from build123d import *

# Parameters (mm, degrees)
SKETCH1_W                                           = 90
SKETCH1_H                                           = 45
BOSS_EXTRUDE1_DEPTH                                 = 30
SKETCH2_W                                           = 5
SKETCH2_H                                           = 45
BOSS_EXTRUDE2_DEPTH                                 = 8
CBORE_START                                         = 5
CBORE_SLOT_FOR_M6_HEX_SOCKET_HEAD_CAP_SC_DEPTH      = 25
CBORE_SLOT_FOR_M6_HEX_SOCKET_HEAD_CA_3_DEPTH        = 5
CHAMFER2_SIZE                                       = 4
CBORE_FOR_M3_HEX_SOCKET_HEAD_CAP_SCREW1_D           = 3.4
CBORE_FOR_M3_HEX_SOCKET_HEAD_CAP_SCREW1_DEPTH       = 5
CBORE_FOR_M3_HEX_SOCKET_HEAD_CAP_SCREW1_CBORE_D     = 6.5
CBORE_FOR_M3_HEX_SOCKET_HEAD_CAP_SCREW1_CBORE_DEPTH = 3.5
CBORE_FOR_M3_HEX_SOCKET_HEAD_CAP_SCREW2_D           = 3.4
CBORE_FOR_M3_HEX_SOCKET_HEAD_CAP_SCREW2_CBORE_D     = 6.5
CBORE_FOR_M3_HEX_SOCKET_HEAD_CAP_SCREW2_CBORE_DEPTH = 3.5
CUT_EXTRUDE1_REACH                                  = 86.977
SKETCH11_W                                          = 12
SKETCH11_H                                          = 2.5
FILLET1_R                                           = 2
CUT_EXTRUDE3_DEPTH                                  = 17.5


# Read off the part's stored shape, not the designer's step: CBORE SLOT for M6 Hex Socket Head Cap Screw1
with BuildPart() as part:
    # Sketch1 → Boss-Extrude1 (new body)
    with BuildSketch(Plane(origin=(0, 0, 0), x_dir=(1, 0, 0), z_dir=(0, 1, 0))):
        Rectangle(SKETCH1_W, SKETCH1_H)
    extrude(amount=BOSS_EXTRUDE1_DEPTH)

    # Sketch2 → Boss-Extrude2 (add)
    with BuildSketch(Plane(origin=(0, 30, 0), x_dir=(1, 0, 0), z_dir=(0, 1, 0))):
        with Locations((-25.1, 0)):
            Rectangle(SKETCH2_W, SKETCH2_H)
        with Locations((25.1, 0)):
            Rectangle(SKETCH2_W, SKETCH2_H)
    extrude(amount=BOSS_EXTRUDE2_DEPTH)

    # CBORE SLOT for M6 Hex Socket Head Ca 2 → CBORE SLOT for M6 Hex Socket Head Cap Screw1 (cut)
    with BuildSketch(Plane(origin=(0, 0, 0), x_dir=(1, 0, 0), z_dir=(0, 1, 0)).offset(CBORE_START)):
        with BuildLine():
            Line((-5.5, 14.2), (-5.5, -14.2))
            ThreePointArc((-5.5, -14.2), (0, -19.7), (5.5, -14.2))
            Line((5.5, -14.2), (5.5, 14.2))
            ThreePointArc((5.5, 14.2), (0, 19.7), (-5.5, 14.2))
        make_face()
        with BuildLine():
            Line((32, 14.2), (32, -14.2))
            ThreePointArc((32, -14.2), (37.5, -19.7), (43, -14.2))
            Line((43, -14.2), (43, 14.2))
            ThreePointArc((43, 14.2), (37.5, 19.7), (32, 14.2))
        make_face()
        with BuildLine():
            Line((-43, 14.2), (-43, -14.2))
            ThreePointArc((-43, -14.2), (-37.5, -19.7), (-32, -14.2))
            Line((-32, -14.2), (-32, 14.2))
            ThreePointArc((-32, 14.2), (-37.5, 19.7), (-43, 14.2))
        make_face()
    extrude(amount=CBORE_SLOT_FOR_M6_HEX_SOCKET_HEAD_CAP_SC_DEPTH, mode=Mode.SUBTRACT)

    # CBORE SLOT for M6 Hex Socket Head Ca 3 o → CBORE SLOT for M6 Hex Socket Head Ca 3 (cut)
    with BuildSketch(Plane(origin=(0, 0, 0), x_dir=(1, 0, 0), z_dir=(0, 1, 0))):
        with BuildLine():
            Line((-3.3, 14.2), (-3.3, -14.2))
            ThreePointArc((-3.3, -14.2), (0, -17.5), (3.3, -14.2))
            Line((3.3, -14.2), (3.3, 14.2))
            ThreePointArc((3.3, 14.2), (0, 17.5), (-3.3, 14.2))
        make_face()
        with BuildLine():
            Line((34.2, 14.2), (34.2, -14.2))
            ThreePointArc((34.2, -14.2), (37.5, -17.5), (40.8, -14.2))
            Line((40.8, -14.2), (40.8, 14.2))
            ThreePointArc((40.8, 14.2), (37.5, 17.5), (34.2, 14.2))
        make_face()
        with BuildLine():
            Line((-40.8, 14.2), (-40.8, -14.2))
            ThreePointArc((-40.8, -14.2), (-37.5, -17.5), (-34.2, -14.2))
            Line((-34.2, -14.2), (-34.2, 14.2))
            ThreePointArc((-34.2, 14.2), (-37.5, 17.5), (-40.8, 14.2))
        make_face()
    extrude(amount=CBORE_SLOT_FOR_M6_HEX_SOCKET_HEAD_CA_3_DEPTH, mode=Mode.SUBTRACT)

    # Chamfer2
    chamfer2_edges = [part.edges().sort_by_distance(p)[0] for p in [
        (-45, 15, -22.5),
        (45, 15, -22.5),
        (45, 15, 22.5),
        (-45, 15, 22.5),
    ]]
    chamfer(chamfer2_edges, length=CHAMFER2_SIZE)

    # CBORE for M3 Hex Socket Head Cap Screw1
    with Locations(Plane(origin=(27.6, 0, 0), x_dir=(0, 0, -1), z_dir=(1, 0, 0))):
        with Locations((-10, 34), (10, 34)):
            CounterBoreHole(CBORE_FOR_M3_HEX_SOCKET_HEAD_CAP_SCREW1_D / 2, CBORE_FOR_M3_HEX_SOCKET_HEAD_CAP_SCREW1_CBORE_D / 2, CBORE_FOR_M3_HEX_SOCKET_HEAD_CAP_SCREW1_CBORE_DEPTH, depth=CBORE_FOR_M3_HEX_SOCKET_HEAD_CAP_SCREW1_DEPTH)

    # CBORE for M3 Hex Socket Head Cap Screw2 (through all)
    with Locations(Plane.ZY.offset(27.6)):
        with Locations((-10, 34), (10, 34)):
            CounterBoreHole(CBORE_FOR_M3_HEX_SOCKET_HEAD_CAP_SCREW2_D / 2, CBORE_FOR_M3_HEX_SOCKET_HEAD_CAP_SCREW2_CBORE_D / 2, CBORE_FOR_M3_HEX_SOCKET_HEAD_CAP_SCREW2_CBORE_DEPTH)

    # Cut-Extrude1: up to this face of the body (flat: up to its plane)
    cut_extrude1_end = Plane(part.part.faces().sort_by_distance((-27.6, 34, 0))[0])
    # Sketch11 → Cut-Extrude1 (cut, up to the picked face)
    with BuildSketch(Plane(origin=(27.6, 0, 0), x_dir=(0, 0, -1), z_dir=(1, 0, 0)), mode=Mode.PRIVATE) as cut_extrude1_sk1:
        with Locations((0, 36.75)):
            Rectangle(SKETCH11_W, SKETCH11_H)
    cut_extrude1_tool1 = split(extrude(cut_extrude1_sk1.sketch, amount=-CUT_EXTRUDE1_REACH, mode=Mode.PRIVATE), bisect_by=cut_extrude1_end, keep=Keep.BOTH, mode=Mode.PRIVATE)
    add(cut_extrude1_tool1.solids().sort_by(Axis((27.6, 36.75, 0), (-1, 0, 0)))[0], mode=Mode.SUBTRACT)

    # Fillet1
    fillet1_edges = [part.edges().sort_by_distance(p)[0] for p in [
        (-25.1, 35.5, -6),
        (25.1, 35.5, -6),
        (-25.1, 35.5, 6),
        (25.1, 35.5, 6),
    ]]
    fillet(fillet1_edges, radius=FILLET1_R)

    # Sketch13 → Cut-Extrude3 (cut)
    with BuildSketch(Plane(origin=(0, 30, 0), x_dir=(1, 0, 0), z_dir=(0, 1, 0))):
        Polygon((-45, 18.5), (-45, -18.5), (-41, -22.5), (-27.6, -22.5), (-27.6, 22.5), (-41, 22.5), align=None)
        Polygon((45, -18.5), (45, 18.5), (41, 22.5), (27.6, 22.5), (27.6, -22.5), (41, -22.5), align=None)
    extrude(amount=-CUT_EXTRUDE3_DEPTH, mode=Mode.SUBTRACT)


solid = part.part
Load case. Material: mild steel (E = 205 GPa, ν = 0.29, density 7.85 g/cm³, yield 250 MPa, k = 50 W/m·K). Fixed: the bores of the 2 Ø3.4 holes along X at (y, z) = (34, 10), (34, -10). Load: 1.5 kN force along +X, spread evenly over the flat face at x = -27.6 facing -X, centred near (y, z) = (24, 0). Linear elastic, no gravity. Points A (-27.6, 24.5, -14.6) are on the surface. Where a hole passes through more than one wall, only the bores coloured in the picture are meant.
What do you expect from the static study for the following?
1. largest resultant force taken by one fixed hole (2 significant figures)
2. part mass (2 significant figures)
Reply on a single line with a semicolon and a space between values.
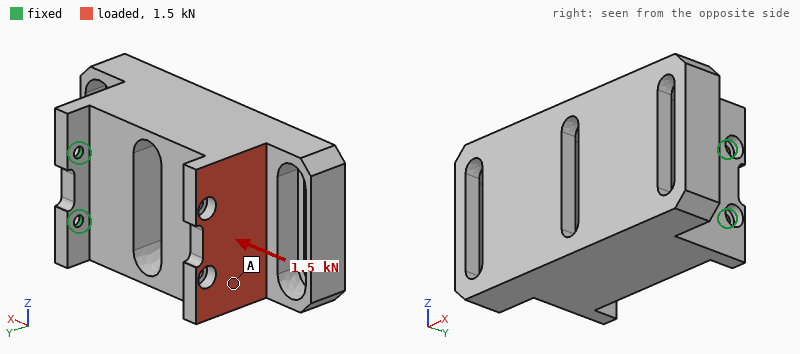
750 N; 600 g
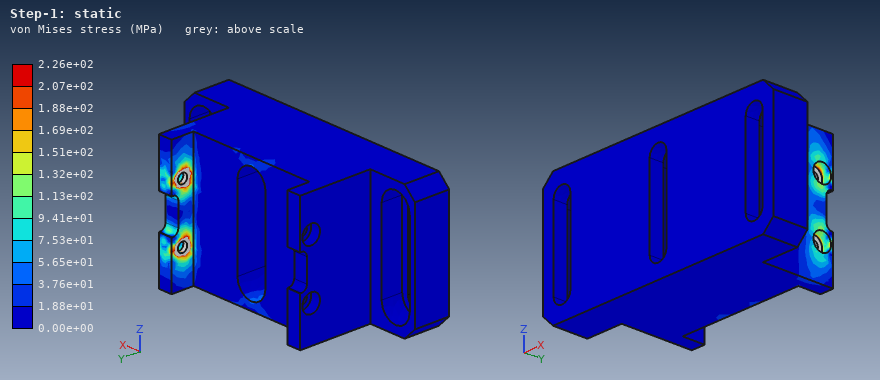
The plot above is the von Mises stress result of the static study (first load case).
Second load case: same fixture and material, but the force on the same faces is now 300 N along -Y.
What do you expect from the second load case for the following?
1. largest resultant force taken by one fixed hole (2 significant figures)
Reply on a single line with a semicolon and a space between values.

150 N
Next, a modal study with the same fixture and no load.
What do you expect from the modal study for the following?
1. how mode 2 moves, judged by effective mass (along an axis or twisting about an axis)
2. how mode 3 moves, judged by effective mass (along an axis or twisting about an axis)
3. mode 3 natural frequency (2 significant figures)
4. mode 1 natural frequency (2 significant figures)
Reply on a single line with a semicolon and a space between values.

along Z; along Z; 3200 Hz; 270 Hz
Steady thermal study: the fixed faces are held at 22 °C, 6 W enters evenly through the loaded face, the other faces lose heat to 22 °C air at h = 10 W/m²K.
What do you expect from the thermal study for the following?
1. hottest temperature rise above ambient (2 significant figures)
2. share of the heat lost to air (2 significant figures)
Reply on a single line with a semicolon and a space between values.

18 K; 35 %
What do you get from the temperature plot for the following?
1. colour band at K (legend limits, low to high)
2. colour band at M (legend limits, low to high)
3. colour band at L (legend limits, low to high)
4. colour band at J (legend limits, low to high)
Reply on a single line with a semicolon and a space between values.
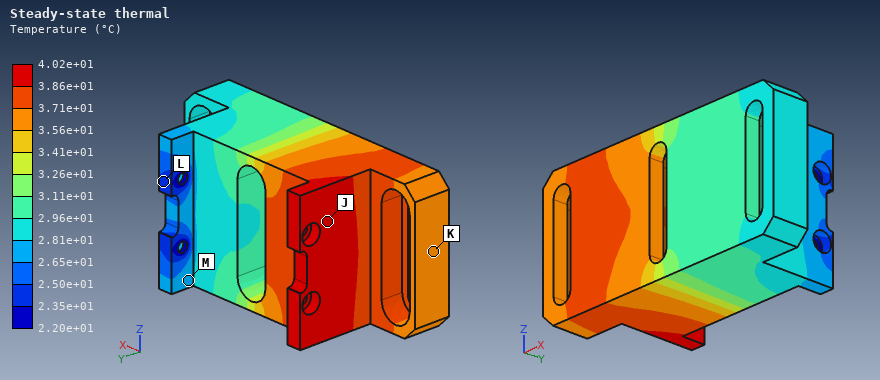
3.56e+01 to 3.71e+01 °C; 2.65e+01 to 2.81e+01 °C; 2.35e+01 to 2.50e+01 °C; 3.86e+01 to 4.02e+01 °C
